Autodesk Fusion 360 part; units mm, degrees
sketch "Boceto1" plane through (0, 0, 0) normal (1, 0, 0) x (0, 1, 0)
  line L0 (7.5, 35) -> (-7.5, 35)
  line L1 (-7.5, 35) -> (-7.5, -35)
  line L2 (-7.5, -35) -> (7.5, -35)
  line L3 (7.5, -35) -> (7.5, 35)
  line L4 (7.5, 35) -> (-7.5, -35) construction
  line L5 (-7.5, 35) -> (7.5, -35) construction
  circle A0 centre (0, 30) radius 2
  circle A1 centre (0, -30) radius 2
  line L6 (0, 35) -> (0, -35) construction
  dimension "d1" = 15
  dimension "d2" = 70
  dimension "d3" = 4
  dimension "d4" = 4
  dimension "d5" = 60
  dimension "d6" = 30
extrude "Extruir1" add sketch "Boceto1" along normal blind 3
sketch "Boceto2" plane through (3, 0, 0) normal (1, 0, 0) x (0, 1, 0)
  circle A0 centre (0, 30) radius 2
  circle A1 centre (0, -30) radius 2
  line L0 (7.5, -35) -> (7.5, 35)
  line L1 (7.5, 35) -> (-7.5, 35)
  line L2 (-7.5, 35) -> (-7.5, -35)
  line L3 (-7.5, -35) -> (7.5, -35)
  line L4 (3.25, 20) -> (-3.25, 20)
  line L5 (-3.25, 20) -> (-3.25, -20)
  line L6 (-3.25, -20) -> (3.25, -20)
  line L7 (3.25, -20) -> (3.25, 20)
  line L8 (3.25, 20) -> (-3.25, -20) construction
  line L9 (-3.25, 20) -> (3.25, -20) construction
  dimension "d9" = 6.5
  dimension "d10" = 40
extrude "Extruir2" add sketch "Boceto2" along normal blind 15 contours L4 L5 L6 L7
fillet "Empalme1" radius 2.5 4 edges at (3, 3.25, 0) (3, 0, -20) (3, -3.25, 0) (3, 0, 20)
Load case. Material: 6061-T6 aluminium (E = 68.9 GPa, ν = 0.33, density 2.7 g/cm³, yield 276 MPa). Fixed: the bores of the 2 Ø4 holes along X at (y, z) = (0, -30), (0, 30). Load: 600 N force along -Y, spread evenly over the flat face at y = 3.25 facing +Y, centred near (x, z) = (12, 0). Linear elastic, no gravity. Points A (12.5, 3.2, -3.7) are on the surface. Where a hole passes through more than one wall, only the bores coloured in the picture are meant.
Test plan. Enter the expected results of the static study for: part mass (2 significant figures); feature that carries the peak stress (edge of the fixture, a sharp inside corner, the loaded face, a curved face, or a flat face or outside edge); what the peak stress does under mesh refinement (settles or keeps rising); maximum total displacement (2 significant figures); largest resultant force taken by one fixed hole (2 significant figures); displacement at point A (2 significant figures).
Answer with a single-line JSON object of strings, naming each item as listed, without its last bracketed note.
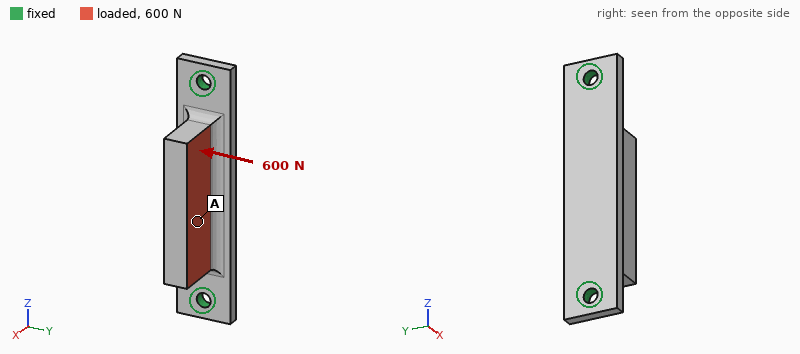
{"part mass": "19 g", "feature that carries the peak stress": "edge of the fixture", "what the peak stress does under mesh refinement": "keeps rising", "maximum total displacement": "0.16 mm", "largest resultant force taken by one fixed hole": "300 N", "displacement at point A": "0.11 mm"}
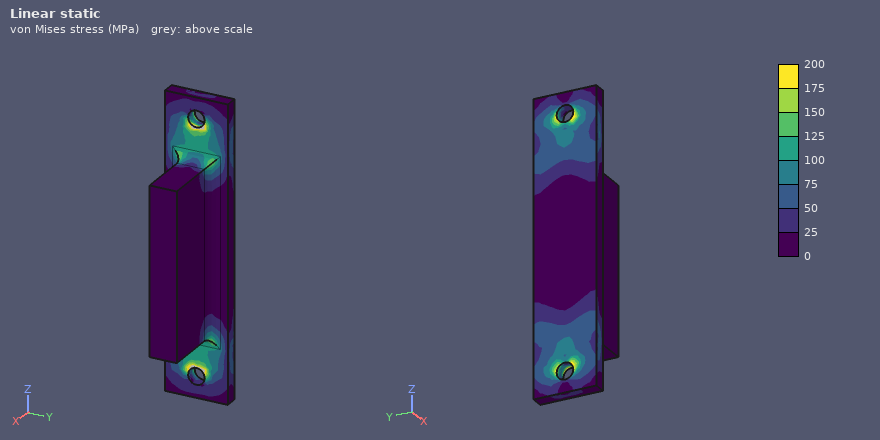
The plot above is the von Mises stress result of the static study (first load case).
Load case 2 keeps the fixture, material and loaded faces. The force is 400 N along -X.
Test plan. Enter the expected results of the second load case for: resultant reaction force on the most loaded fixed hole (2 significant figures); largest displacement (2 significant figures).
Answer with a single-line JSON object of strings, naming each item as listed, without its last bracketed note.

{"resultant reaction force on the most loaded fixed hole": "250 N", "largest displacement": "36 µm"}
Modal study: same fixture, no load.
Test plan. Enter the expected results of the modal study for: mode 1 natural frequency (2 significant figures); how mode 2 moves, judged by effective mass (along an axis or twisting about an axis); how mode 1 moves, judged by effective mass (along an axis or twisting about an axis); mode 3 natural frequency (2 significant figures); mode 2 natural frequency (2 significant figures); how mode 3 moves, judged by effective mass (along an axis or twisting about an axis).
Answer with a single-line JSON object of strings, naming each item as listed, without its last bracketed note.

{"mode 1 natural frequency": "3800 Hz", "how mode 2 moves, judged by effective mass": "along X", "how mode 1 moves, judged by effective mass": "along Y", "mode 3 natural frequency": "11 kHz", "mode 2 natural frequency": "7100 Hz", "how mode 3 moves, judged by effective mass": "along Y"}
